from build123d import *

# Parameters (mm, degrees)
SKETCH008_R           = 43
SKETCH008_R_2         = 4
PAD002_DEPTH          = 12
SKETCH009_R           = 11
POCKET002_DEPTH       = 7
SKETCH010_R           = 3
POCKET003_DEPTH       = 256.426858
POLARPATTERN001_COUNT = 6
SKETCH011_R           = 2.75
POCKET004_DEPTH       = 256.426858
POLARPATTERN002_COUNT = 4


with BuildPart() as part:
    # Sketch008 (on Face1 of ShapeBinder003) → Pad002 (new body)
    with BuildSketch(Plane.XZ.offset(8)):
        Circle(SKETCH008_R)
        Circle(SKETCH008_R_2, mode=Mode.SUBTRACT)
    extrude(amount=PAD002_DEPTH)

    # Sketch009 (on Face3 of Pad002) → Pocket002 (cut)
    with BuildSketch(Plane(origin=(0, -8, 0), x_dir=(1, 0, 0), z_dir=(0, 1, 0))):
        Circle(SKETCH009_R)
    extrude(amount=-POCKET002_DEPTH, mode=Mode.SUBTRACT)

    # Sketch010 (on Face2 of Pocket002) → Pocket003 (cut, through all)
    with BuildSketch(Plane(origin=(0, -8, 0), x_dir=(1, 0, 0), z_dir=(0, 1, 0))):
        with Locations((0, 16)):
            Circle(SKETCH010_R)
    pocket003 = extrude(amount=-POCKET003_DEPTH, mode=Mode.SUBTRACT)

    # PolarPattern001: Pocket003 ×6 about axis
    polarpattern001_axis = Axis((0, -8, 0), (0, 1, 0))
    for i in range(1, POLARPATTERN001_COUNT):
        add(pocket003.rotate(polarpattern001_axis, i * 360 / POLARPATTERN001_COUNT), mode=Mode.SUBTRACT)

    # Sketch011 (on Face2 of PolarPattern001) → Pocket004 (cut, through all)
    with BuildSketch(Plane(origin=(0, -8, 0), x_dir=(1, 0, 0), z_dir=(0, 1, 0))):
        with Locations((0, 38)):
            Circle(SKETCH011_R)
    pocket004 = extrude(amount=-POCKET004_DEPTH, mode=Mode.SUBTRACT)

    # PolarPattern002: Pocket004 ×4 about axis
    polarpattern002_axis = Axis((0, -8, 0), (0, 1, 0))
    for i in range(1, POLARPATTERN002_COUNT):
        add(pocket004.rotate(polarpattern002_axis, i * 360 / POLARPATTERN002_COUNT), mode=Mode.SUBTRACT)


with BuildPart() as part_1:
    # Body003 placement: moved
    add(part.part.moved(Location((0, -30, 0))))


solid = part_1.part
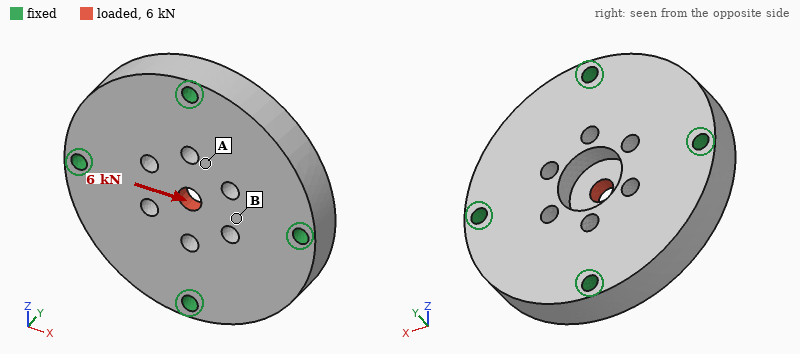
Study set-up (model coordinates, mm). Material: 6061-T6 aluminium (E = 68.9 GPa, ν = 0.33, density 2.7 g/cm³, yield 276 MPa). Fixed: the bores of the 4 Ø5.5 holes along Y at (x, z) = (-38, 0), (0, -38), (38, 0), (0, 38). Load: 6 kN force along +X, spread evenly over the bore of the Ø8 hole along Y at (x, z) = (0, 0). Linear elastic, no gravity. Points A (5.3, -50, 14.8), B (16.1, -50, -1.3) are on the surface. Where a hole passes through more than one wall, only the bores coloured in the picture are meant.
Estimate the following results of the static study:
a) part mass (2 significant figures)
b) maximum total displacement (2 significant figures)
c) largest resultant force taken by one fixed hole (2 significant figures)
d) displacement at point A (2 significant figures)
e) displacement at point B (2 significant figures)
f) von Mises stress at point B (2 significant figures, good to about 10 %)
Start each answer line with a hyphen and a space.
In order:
- 170 g
- 11 µm
- 2.0 kN
- 3.5 µm
- 4.8 µm
- 22 MPa
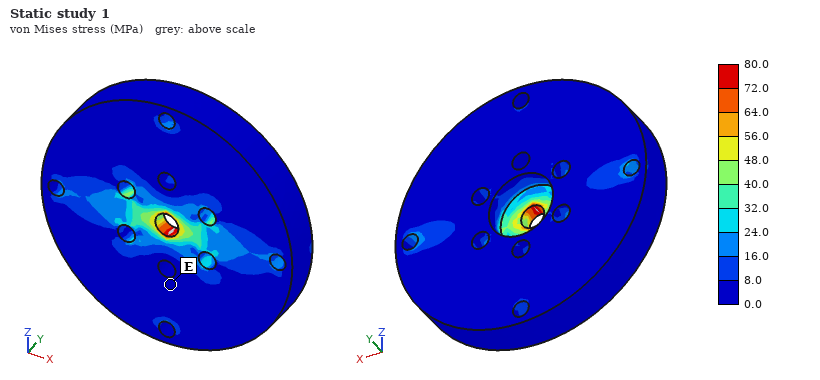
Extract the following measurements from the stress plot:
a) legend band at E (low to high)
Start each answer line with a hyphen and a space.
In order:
- 0.0 to 8.0 MPa
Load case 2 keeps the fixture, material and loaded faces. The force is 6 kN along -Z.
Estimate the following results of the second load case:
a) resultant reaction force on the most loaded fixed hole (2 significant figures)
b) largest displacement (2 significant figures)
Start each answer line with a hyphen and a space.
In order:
- 2.0 kN
- 11 µm
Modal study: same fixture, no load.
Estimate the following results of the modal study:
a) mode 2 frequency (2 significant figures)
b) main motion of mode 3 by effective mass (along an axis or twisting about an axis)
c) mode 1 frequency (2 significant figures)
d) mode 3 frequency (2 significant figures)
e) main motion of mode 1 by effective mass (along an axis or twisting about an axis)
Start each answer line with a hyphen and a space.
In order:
- 14 kHz
- twisting about Z
- 12 kHz
- 15 kHz
- along Y
